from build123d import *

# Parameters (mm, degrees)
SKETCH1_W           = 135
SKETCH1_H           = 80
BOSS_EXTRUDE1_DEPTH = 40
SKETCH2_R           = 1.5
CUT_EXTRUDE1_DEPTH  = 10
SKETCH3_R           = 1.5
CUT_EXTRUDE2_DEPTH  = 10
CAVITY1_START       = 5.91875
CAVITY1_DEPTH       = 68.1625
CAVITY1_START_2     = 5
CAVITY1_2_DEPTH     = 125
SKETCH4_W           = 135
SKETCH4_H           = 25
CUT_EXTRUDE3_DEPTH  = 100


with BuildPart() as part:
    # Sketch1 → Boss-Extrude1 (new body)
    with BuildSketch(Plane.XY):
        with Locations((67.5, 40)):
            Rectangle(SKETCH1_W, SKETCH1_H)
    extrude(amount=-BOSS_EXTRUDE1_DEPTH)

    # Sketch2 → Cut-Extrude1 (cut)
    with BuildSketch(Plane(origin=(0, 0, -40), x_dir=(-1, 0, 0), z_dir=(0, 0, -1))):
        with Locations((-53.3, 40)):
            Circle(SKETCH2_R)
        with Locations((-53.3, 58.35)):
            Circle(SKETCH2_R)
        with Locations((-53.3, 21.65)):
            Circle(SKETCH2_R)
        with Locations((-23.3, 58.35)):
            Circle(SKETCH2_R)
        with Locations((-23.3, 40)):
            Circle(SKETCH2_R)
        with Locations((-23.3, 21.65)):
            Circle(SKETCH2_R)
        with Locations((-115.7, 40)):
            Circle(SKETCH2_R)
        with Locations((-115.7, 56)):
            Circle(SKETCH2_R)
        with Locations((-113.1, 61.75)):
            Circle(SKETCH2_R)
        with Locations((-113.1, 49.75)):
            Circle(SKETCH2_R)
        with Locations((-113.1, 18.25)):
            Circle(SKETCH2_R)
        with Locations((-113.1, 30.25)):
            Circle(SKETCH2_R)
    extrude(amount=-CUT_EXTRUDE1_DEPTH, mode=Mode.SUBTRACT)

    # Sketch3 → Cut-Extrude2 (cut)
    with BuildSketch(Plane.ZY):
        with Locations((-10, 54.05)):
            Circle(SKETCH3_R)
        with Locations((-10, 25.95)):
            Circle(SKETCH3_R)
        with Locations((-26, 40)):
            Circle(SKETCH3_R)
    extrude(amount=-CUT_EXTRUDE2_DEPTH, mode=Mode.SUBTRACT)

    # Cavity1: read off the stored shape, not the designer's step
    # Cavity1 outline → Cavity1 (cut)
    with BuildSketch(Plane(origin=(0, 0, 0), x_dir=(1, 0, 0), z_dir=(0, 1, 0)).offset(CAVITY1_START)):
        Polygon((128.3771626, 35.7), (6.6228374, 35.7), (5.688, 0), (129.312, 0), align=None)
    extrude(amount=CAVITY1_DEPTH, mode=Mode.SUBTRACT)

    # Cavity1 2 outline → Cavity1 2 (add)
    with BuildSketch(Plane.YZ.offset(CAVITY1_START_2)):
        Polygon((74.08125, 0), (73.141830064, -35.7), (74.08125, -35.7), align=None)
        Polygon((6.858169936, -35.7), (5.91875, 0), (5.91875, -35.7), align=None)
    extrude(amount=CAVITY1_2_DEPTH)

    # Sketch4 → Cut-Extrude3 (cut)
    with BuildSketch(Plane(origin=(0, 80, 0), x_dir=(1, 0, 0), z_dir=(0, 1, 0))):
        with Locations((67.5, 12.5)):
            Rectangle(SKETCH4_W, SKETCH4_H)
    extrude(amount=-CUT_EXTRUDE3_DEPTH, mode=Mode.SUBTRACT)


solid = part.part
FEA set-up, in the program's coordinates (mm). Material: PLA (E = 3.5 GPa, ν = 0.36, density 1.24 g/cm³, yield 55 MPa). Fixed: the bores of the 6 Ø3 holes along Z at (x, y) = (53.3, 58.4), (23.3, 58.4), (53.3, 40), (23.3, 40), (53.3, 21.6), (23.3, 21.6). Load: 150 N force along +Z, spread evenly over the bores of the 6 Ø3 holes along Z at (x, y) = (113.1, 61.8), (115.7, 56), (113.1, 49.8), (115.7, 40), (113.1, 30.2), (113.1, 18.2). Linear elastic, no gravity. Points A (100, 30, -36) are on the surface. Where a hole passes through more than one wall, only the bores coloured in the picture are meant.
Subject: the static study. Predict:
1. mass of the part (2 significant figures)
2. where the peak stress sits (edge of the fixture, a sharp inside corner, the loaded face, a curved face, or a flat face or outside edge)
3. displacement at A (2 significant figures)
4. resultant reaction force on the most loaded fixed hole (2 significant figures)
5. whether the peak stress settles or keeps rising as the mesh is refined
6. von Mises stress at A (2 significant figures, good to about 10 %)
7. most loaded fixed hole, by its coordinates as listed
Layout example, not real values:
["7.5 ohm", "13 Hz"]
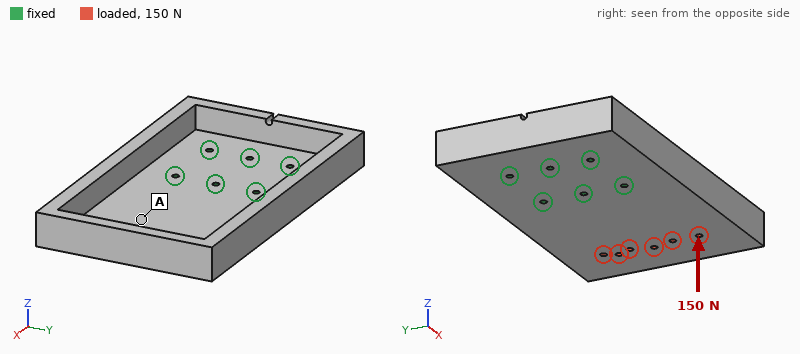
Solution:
["93 g", "edge of the fixture", "0.95 mm", "200 N", "keeps rising", "2.3 MPa", "(53.3, 58.4)"]
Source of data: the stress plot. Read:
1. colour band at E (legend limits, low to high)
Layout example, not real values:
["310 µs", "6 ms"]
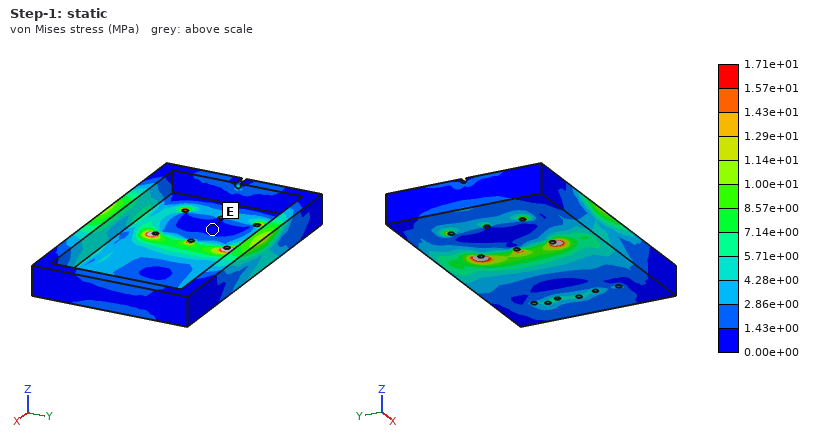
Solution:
["0.00e+00 to 1.43e+00 MPa"]
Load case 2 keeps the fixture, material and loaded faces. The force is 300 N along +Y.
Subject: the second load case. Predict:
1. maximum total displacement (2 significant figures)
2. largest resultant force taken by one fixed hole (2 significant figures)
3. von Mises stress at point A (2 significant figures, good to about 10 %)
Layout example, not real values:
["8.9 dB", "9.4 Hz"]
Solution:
["0.20 mm", "280 N", "2.4 MPa"]
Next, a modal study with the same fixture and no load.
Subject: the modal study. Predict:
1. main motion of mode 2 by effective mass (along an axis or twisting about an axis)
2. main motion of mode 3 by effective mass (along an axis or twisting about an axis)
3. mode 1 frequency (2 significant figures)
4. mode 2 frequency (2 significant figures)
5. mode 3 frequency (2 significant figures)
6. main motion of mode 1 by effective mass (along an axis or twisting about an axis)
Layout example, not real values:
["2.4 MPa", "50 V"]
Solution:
["twisting about X", "along Y", "270 Hz", "420 Hz", "1200 Hz", "along Z"]
